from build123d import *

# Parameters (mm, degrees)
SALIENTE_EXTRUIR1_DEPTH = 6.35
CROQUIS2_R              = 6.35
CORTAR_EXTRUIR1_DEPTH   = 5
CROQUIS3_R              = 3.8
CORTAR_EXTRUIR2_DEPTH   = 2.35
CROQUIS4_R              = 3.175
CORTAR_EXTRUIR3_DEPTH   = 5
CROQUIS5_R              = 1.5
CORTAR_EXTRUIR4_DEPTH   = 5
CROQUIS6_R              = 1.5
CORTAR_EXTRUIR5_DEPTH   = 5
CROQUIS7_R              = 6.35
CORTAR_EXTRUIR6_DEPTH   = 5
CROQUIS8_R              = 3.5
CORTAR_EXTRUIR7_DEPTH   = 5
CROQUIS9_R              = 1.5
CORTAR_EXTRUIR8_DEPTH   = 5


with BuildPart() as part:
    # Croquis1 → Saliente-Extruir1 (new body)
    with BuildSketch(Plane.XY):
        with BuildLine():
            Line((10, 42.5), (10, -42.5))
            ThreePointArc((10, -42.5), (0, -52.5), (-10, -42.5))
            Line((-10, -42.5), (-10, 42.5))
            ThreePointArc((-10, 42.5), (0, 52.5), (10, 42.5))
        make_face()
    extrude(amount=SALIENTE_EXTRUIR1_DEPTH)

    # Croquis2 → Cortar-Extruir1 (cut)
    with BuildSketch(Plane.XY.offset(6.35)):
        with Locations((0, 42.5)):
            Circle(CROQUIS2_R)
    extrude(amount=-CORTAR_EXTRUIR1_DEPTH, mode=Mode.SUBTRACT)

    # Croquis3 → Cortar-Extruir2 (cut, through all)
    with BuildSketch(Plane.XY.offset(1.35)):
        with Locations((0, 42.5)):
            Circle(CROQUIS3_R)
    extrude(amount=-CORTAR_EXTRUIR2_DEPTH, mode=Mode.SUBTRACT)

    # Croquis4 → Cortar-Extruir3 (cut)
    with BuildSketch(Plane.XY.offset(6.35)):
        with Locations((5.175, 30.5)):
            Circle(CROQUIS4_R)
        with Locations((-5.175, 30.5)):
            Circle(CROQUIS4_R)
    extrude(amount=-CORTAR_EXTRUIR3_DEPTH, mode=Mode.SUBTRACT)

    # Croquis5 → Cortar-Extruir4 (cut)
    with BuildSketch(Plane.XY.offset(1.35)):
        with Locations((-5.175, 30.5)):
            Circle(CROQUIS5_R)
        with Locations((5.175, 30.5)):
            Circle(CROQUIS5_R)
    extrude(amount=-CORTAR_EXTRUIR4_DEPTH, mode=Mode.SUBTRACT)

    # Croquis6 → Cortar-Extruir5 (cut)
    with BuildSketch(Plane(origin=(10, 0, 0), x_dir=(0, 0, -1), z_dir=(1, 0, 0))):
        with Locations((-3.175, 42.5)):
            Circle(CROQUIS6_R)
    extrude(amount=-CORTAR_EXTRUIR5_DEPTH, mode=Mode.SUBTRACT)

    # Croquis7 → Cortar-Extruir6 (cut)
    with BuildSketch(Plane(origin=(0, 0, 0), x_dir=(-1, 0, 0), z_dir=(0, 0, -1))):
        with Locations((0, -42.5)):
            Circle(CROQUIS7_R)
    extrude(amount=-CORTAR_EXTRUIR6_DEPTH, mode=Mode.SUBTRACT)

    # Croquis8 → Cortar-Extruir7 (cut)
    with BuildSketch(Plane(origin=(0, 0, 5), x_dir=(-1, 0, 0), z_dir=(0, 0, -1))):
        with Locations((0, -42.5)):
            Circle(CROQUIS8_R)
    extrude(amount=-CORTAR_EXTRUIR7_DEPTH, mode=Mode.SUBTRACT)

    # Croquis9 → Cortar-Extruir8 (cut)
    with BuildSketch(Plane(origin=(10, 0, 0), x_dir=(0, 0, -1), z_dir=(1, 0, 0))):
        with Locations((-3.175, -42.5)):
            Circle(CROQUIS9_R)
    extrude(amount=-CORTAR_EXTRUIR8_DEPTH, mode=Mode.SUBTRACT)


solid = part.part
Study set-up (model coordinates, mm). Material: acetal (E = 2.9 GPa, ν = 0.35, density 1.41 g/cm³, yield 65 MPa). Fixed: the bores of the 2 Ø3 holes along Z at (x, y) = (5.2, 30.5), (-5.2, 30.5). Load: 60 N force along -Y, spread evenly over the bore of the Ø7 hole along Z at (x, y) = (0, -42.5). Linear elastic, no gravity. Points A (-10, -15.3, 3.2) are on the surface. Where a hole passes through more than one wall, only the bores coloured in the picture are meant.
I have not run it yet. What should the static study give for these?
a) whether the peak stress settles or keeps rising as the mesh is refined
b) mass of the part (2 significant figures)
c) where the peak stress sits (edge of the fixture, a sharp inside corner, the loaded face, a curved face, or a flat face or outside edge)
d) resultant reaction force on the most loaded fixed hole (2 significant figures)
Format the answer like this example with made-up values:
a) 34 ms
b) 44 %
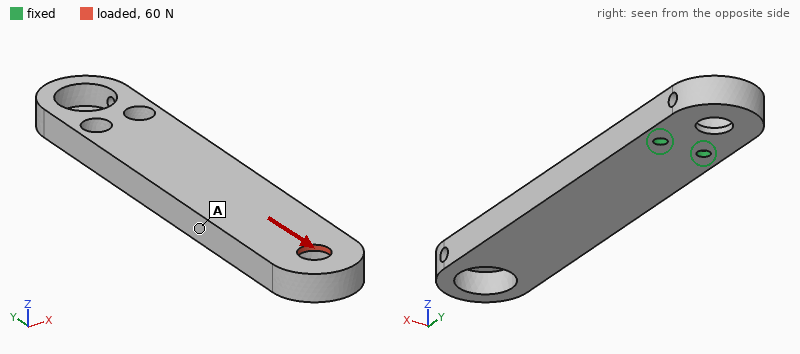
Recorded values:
a) keeps rising
b) 16 g
c) edge of the fixture
d) 30 N
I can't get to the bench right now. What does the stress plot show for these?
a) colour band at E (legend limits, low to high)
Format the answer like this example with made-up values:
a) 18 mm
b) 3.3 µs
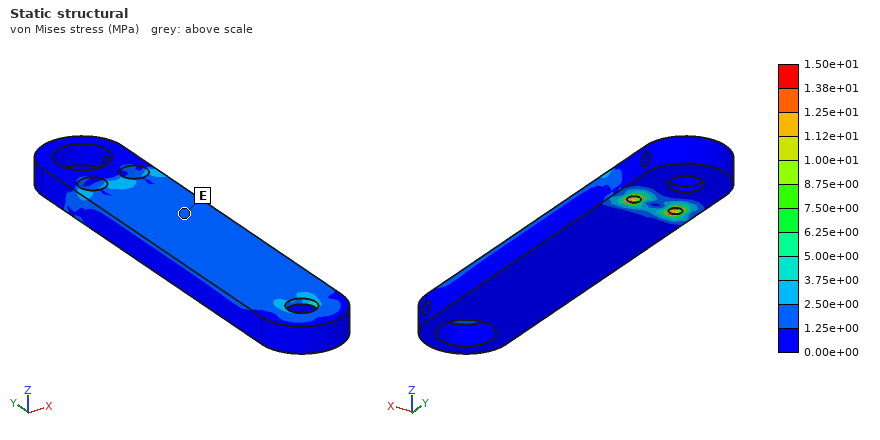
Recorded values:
a) 1.25e+00 to 2.50e+00 MPa
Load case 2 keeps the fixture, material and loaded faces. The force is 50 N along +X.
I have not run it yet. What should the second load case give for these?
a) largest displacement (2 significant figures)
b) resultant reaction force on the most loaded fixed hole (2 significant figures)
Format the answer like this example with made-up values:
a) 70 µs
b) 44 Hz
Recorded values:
a) 1.1 mm
b) 310 N
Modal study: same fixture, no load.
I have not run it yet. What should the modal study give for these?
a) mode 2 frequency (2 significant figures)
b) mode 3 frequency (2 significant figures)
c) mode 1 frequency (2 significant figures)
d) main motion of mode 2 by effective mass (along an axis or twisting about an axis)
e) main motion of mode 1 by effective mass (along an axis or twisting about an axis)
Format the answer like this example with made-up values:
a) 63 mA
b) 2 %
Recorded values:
a) 550 Hz
b) 1100 Hz
c) 140 Hz
d) along X
e) along Z
